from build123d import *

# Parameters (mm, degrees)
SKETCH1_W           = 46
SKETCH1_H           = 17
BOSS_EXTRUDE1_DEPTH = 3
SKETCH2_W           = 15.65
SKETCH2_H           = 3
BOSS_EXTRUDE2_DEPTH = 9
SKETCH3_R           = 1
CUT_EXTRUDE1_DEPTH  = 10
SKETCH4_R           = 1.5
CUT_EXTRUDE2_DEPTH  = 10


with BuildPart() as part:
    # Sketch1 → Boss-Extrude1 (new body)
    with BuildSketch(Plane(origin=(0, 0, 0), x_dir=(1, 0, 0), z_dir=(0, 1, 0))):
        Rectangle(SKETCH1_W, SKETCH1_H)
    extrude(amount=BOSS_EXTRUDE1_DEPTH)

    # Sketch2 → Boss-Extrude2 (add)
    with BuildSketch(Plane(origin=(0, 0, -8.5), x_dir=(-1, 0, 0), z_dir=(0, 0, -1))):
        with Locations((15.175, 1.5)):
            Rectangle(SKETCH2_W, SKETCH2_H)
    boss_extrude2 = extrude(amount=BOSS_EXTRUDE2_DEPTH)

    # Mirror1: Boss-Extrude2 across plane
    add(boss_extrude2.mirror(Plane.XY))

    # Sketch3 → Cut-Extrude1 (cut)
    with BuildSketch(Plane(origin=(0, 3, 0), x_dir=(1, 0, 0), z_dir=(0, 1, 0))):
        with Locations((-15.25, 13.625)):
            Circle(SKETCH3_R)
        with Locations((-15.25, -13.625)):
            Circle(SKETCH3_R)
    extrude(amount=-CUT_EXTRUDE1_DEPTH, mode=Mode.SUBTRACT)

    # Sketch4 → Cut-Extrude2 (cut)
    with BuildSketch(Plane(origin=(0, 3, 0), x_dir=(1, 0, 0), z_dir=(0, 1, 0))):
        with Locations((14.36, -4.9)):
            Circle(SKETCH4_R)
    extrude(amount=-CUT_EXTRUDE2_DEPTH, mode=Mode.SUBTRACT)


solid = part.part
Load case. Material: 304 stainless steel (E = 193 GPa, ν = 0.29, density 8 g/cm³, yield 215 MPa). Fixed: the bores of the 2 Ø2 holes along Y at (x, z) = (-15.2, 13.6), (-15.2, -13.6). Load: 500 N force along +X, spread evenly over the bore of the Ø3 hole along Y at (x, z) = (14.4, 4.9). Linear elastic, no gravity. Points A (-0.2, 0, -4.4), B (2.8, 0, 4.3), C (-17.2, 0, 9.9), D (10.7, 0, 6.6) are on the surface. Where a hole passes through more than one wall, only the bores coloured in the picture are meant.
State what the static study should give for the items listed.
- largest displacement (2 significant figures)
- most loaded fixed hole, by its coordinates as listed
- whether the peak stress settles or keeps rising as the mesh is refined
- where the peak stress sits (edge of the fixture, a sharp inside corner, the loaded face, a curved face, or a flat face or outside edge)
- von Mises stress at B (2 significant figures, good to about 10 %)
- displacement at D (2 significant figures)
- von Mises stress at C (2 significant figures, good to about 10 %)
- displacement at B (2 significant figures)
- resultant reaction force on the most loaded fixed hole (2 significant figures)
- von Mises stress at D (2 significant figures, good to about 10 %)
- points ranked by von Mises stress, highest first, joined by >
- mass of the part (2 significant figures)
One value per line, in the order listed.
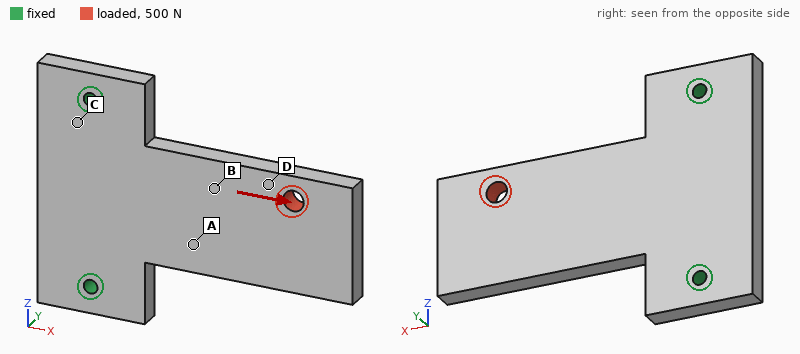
7.9 µm
(-15.2, 13.6)
keeps rising
edge of the fixture
18 MPa
4.7 µm
13 MPa
2.6 µm
350 N
24 MPa
D > B > C > A
25 g
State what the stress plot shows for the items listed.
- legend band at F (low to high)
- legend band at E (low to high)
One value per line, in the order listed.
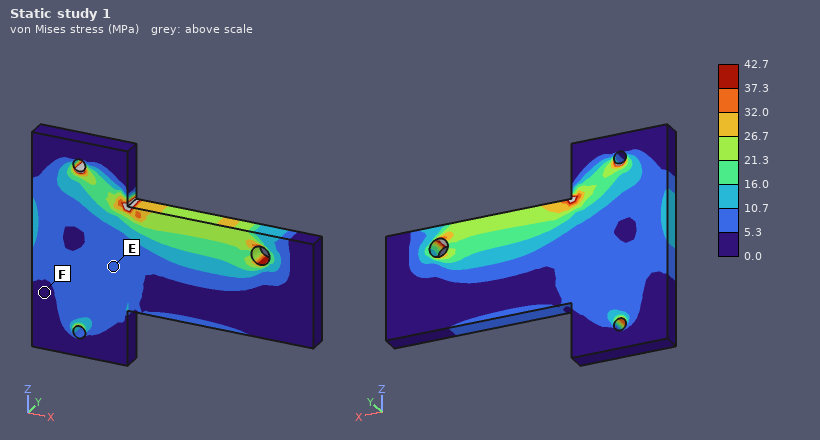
0.0 to 5.3 MPa
5.3 to 10.7 MPa
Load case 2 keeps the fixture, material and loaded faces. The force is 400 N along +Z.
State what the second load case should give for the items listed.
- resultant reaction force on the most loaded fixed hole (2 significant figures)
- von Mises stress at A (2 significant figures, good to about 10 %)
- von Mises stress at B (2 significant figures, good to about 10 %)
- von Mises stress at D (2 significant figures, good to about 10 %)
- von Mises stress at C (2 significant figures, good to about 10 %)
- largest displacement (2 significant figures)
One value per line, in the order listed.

480 N
26 MPa
22 MPa
12 MPa
12 MPa
20 µm
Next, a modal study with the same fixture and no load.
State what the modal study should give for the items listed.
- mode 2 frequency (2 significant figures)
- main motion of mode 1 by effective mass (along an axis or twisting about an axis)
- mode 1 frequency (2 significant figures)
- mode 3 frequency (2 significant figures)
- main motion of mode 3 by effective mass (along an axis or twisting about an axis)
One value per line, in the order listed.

7800 Hz
along Y
1600 Hz
8900 Hz
along Y
